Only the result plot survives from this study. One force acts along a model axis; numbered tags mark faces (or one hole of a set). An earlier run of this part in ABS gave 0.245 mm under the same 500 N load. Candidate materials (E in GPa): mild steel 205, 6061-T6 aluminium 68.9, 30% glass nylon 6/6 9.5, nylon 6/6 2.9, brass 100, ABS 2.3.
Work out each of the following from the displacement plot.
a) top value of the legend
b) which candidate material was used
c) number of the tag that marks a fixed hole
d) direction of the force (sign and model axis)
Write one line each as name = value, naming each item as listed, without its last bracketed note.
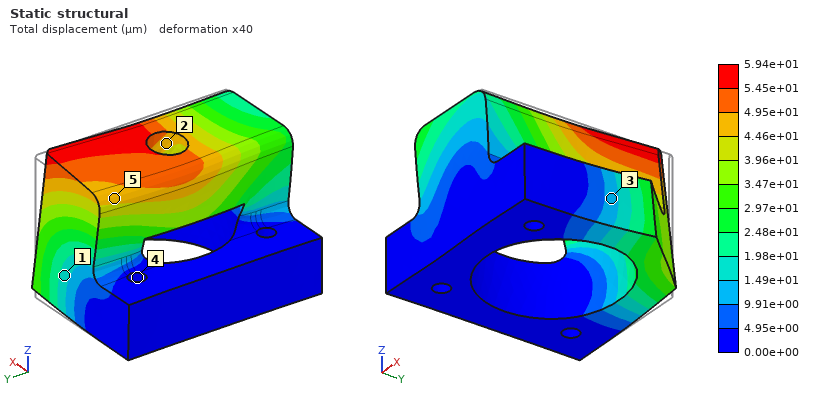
top value of the legend = 5.94e+01 µm
which candidate material was used = 30% glass nylon 6/6
number of the tag that marks a fixed hole = 4
direction of the force = -X
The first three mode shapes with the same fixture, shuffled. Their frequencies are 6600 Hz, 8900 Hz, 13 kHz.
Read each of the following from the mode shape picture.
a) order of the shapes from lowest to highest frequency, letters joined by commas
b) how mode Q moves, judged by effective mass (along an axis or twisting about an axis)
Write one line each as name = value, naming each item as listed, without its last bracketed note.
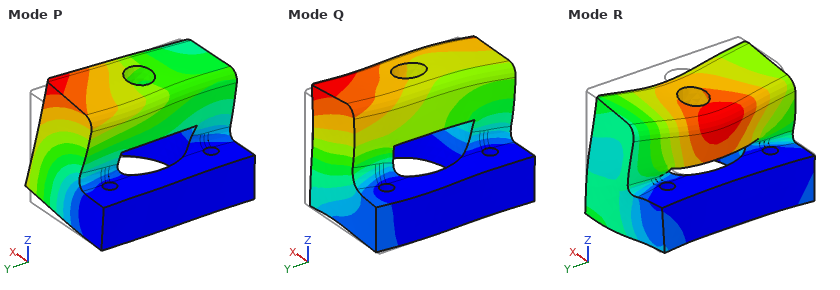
order of the shapes from lowest to highest frequency, letters joined by commas = P, Q, R
how mode Q moves, judged by effective mass = along Y
